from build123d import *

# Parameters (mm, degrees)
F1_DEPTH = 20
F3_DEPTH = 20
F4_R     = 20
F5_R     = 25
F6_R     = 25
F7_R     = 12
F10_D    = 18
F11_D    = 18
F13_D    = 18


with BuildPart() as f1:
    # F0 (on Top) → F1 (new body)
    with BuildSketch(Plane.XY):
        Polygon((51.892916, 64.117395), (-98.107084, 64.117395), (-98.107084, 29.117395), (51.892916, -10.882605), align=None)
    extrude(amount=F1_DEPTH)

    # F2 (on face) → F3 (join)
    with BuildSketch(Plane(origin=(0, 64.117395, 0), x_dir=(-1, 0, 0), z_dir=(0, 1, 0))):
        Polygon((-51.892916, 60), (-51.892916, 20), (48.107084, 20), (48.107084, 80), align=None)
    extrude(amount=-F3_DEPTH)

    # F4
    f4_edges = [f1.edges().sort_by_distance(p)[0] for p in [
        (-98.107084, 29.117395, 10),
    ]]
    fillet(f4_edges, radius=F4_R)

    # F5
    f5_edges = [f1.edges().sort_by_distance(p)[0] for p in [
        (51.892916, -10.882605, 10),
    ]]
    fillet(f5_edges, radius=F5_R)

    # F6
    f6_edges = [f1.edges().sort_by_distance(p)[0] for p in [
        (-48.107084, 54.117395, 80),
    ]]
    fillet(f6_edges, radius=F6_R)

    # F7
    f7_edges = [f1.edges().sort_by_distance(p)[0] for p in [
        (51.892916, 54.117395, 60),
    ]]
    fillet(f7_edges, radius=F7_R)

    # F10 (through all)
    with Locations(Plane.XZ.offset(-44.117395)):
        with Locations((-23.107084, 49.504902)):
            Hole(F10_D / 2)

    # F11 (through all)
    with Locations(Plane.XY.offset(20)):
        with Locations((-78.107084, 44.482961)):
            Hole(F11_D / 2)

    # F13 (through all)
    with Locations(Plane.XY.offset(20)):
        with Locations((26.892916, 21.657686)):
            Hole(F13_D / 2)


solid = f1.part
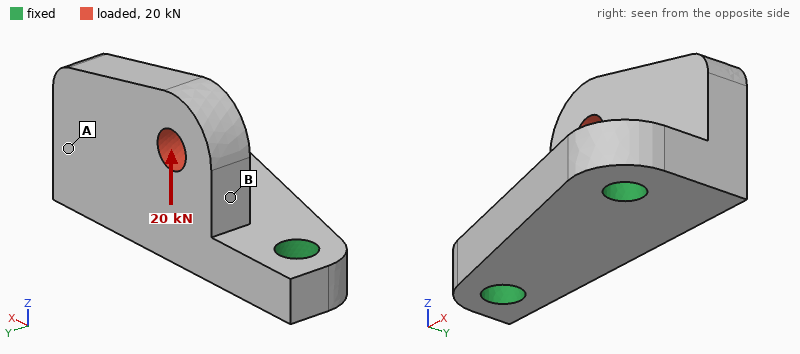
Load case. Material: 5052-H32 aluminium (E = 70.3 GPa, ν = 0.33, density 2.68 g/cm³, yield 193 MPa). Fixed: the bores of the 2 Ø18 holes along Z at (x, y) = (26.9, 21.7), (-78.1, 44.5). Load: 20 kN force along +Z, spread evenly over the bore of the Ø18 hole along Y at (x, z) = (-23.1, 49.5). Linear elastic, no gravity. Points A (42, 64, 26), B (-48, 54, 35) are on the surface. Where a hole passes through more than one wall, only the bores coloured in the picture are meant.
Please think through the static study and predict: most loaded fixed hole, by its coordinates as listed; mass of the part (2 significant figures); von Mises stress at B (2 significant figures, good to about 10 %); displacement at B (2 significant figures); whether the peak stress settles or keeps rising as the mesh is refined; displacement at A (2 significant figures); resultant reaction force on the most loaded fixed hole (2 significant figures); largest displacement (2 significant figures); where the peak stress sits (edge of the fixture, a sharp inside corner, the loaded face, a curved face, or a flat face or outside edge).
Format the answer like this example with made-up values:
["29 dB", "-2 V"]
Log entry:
["(-78.1, 44.5)", "640 g", "33 MPa", "0.075 mm", "keeps rising", "0.047 mm", "11 kN", "0.13 mm", "edge of the fixture"]
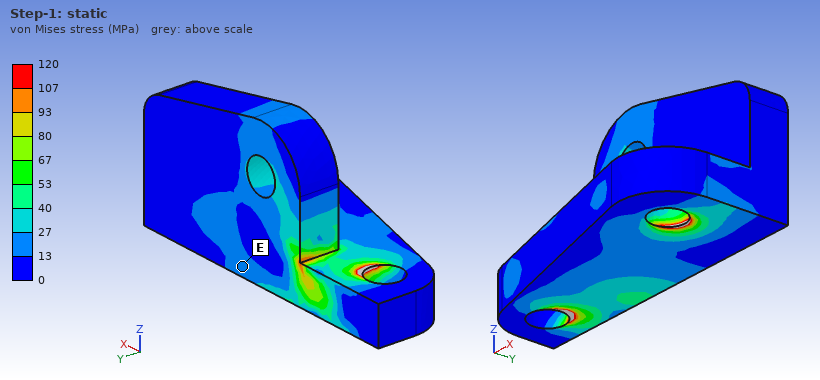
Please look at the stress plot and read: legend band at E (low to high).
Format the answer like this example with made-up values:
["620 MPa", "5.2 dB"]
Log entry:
["13 to 27 MPa"]
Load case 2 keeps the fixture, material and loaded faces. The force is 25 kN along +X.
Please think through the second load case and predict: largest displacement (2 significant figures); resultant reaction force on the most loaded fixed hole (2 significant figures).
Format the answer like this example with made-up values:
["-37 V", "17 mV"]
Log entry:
["0.11 mm", "17 kN"]
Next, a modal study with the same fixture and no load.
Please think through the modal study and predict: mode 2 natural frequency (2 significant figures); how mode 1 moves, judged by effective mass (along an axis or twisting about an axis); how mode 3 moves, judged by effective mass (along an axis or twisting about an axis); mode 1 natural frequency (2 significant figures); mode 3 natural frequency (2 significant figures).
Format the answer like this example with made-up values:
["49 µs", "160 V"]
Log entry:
["5600 Hz", "along Y", "along Z", "2800 Hz", "6400 Hz"]
